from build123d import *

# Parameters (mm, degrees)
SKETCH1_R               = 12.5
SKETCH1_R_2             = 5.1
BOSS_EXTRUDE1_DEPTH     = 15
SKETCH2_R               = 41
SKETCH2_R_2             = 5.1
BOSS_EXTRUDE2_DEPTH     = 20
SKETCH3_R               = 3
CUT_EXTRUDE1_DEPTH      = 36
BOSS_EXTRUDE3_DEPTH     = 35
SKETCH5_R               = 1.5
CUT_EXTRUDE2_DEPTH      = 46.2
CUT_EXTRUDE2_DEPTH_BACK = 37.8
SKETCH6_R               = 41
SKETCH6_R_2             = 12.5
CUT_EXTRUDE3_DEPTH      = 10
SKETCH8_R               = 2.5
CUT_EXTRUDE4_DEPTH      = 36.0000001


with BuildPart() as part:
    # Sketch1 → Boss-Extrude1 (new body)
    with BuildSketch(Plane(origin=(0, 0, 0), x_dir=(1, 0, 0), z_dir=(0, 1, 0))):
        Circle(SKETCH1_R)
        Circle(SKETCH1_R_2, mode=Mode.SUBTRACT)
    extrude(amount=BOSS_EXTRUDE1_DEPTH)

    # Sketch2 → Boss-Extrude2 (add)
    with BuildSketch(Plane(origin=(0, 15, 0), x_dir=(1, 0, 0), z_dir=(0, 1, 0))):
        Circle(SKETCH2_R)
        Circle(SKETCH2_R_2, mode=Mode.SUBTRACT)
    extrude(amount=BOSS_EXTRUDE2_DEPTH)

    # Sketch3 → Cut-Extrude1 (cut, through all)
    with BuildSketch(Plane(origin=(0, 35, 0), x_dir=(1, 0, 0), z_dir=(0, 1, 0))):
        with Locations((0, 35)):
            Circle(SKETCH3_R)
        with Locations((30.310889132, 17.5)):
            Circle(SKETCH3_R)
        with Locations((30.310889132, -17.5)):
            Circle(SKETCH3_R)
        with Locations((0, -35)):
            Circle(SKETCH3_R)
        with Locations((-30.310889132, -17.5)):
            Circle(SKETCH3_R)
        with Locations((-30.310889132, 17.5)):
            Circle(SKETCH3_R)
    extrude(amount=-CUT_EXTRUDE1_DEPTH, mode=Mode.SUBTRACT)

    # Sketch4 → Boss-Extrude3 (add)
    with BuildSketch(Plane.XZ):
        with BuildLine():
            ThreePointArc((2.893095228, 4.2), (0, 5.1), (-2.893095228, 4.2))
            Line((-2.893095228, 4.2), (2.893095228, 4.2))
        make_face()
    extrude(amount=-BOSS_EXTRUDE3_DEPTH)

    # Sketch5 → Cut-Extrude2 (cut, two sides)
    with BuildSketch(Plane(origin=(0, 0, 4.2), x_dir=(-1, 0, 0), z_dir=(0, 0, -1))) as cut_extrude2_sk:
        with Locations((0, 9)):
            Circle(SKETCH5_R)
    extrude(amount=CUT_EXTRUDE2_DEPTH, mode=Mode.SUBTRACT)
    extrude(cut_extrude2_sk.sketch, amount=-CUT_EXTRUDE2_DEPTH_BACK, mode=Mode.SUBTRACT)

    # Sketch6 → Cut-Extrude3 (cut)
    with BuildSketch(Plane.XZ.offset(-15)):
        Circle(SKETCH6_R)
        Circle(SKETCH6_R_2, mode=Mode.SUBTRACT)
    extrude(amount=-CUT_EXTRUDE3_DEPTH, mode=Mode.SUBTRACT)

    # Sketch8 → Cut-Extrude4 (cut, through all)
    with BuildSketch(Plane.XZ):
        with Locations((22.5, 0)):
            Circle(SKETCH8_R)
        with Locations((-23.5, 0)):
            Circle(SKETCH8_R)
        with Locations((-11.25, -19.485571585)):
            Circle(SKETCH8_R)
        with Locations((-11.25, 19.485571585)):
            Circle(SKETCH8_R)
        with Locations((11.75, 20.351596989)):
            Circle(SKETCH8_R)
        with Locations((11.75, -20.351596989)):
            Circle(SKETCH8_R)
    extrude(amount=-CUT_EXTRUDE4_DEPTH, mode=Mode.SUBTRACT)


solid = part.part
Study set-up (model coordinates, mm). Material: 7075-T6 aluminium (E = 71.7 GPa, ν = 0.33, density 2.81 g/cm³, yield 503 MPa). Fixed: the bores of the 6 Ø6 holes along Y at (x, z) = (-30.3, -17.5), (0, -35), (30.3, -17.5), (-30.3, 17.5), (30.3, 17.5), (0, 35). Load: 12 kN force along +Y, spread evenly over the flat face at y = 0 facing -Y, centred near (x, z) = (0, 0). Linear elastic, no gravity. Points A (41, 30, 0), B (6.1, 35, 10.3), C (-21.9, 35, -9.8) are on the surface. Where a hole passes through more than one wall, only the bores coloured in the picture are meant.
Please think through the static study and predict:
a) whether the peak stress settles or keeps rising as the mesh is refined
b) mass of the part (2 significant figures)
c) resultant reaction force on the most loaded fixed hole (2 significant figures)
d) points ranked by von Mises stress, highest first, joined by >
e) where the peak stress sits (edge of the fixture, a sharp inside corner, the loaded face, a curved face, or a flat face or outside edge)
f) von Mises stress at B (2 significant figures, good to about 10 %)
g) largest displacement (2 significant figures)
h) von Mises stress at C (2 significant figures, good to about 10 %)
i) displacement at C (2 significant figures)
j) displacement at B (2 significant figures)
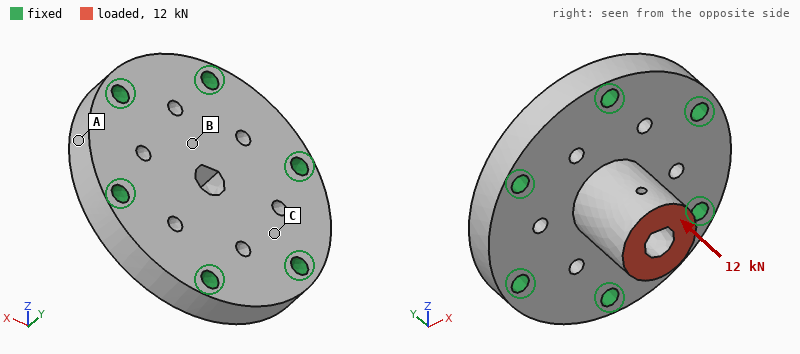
keeps rising
170 g
2.1 kN
B > C > A
edge of the fixture
47 MPa
47 µm
25 MPa
15 µm
34 µm
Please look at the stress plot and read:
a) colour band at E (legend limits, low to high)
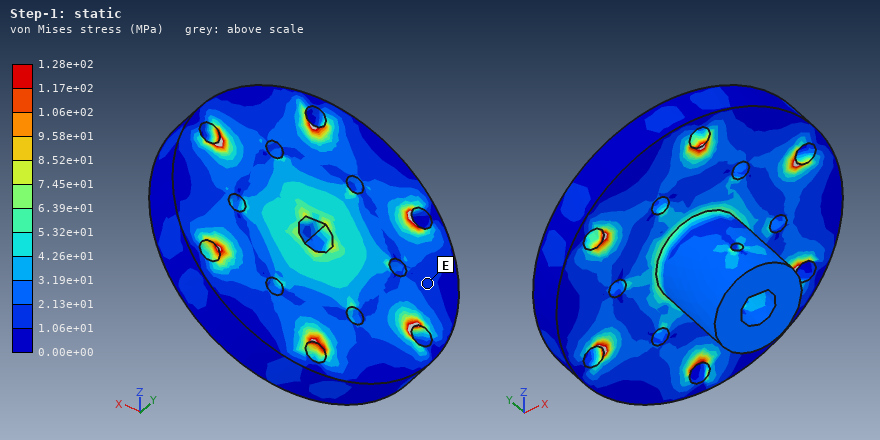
1.06e+01 to 2.13e+01 MPa
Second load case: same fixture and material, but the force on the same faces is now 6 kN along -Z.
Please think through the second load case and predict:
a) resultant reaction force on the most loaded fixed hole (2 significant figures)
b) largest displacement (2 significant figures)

2.7 kN
0.11 mm
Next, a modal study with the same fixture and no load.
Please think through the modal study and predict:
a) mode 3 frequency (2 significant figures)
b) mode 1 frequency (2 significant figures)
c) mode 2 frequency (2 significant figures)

12 kHz
11 kHz
11 kHz
